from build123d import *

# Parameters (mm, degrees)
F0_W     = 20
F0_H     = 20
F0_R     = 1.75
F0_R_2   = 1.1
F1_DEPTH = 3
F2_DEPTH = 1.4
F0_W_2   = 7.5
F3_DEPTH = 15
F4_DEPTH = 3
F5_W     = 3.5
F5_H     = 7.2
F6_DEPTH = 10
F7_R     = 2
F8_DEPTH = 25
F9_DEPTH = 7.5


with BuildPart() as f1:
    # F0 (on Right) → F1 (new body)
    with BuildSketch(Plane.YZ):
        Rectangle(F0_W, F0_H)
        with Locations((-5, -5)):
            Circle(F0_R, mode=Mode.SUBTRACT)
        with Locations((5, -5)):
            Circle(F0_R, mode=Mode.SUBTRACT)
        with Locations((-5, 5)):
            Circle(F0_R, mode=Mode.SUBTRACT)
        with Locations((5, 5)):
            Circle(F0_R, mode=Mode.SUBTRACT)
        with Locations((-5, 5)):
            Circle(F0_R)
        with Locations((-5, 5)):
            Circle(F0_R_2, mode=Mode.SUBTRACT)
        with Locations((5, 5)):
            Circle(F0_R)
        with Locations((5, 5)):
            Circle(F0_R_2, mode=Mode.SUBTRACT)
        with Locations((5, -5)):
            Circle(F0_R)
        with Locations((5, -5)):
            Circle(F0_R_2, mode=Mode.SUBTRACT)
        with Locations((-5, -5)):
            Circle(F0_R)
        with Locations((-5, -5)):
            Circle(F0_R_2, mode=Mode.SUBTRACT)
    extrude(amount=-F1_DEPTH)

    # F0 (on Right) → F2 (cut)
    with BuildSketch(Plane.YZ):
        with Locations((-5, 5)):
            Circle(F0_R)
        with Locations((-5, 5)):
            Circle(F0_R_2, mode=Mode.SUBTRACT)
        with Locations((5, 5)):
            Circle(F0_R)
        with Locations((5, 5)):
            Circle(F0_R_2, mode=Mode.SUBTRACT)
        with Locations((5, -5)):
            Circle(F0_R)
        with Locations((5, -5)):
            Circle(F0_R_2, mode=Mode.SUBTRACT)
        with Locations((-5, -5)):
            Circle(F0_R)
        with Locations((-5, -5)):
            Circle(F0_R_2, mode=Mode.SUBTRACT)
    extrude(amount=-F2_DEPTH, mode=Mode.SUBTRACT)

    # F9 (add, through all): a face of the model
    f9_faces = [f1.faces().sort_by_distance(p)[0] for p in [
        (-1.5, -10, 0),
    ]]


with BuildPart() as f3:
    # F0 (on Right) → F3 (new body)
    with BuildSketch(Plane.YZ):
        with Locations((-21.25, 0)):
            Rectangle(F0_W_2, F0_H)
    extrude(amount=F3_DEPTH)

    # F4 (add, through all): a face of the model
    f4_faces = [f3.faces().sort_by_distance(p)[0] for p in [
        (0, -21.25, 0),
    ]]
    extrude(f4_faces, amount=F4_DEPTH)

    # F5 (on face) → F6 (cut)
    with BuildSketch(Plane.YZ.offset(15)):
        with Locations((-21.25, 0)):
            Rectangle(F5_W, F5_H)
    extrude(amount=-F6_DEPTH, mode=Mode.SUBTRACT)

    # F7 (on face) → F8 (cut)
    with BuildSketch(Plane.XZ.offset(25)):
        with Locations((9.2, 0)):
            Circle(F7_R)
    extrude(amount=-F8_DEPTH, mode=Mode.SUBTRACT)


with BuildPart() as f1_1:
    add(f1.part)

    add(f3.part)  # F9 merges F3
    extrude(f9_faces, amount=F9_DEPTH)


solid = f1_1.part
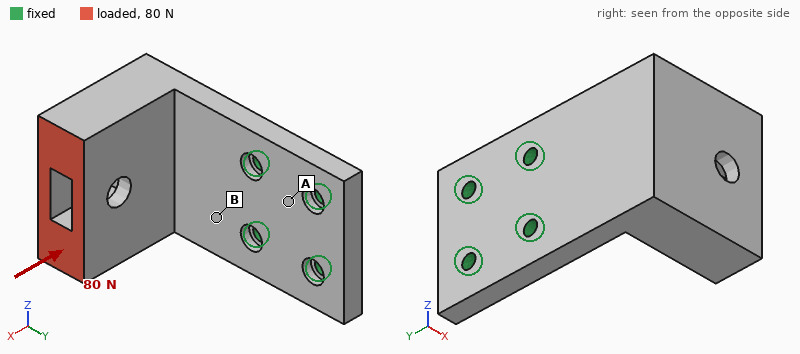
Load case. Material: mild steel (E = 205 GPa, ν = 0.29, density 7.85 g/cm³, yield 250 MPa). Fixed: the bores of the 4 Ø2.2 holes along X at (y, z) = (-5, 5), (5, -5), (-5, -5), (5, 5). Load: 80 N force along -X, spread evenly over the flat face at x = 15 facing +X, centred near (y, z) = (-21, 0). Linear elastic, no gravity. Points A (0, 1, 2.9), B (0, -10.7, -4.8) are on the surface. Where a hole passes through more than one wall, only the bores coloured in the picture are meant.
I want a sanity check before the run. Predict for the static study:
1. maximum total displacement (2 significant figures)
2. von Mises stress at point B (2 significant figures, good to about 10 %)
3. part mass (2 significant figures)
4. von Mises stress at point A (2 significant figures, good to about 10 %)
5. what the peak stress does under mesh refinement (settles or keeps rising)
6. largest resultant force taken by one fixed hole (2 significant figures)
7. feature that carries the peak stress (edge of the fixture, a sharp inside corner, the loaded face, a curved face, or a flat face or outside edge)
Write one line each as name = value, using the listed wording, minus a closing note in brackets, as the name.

maximum total displacement = 31 µm
von Mises stress at point B = 23 MPa
part mass = 31 g
von Mises stress at point A = 6.8 MPa
what the peak stress does under mesh refinement = keeps rising
largest resultant force taken by one fixed hole = 100 N
feature that carries the peak stress = edge of the fixture
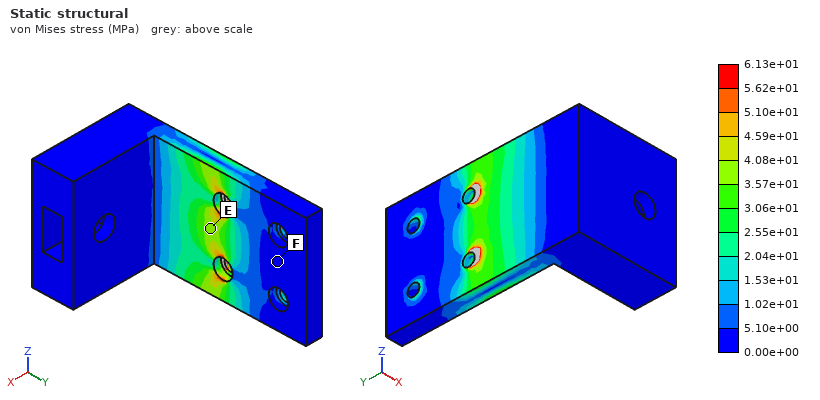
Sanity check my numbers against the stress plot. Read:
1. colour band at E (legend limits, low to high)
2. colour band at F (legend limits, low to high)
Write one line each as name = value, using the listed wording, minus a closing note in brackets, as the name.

colour band at E = 3.57e+01 to 4.08e+01 MPa
colour band at F = 0.00e+00 to 5.10e+00 MPa
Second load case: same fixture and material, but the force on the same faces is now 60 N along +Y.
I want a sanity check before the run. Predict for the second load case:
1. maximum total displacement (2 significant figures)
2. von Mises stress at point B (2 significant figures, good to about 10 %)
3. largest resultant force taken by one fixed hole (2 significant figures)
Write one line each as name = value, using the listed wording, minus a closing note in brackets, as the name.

maximum total displacement = 37 µm
von Mises stress at point B = 29 MPa
largest resultant force taken by one fixed hole = 70 N
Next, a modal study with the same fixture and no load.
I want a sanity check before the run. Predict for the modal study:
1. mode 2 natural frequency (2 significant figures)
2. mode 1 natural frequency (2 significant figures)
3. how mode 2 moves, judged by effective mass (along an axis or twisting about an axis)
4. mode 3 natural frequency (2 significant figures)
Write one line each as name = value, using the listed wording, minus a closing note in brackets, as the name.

mode 2 natural frequency = 4300 Hz
mode 1 natural frequency = 2000 Hz
how mode 2 moves, judged by effective mass = along Z
mode 3 natural frequency = 9000 Hz
